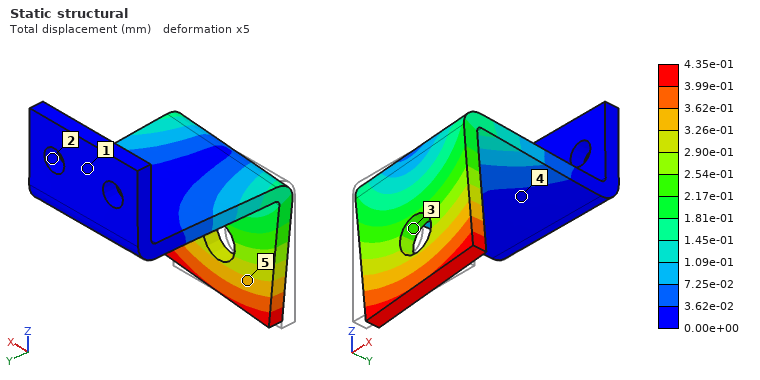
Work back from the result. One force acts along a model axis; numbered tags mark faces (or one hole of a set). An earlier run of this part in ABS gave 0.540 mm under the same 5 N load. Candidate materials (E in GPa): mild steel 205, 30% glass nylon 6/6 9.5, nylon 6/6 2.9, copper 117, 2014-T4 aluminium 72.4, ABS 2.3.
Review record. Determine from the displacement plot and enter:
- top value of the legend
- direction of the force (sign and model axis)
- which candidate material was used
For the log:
4.35e-01 mm
+X
nylon 6/6
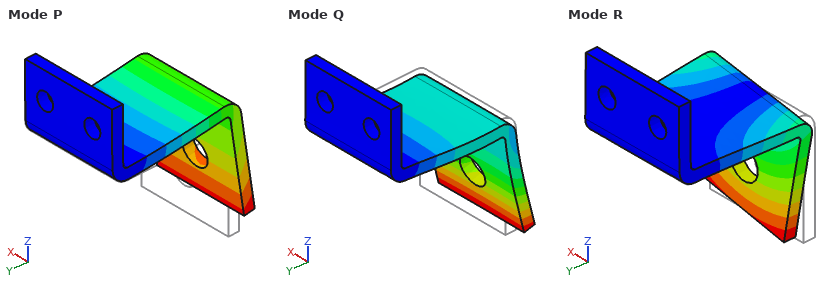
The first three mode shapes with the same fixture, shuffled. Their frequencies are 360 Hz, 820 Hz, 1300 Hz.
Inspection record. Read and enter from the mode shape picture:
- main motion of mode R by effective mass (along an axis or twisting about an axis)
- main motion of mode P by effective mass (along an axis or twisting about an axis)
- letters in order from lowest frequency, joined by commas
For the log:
along X
along Z
P, R, Q
